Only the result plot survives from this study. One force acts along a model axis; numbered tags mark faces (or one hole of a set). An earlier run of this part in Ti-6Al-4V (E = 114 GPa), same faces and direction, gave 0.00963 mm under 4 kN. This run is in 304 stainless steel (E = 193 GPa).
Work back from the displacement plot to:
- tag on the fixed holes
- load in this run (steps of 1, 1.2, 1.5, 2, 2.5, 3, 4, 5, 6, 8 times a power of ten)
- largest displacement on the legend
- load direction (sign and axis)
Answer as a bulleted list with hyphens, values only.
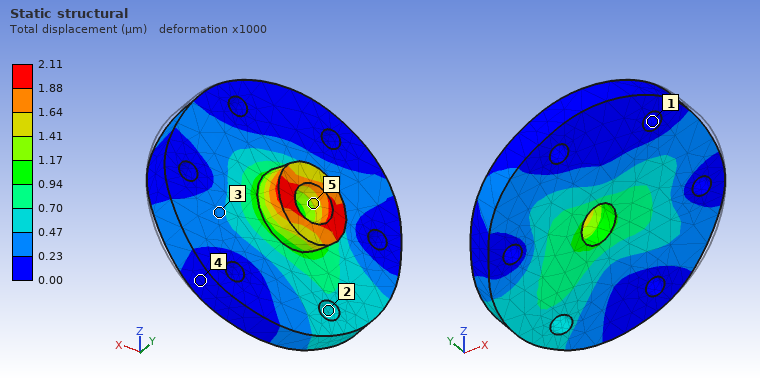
- 1
- 1.5 kN
- 2.11 µm
- -X
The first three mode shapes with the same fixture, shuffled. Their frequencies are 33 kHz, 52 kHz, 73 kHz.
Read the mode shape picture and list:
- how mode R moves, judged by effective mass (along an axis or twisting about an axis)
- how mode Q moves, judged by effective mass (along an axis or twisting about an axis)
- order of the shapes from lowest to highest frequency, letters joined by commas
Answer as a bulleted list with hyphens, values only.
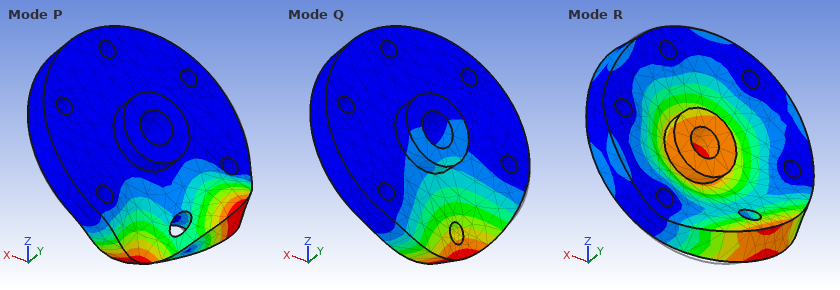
- along Y
- along Y
- Q, R, P
